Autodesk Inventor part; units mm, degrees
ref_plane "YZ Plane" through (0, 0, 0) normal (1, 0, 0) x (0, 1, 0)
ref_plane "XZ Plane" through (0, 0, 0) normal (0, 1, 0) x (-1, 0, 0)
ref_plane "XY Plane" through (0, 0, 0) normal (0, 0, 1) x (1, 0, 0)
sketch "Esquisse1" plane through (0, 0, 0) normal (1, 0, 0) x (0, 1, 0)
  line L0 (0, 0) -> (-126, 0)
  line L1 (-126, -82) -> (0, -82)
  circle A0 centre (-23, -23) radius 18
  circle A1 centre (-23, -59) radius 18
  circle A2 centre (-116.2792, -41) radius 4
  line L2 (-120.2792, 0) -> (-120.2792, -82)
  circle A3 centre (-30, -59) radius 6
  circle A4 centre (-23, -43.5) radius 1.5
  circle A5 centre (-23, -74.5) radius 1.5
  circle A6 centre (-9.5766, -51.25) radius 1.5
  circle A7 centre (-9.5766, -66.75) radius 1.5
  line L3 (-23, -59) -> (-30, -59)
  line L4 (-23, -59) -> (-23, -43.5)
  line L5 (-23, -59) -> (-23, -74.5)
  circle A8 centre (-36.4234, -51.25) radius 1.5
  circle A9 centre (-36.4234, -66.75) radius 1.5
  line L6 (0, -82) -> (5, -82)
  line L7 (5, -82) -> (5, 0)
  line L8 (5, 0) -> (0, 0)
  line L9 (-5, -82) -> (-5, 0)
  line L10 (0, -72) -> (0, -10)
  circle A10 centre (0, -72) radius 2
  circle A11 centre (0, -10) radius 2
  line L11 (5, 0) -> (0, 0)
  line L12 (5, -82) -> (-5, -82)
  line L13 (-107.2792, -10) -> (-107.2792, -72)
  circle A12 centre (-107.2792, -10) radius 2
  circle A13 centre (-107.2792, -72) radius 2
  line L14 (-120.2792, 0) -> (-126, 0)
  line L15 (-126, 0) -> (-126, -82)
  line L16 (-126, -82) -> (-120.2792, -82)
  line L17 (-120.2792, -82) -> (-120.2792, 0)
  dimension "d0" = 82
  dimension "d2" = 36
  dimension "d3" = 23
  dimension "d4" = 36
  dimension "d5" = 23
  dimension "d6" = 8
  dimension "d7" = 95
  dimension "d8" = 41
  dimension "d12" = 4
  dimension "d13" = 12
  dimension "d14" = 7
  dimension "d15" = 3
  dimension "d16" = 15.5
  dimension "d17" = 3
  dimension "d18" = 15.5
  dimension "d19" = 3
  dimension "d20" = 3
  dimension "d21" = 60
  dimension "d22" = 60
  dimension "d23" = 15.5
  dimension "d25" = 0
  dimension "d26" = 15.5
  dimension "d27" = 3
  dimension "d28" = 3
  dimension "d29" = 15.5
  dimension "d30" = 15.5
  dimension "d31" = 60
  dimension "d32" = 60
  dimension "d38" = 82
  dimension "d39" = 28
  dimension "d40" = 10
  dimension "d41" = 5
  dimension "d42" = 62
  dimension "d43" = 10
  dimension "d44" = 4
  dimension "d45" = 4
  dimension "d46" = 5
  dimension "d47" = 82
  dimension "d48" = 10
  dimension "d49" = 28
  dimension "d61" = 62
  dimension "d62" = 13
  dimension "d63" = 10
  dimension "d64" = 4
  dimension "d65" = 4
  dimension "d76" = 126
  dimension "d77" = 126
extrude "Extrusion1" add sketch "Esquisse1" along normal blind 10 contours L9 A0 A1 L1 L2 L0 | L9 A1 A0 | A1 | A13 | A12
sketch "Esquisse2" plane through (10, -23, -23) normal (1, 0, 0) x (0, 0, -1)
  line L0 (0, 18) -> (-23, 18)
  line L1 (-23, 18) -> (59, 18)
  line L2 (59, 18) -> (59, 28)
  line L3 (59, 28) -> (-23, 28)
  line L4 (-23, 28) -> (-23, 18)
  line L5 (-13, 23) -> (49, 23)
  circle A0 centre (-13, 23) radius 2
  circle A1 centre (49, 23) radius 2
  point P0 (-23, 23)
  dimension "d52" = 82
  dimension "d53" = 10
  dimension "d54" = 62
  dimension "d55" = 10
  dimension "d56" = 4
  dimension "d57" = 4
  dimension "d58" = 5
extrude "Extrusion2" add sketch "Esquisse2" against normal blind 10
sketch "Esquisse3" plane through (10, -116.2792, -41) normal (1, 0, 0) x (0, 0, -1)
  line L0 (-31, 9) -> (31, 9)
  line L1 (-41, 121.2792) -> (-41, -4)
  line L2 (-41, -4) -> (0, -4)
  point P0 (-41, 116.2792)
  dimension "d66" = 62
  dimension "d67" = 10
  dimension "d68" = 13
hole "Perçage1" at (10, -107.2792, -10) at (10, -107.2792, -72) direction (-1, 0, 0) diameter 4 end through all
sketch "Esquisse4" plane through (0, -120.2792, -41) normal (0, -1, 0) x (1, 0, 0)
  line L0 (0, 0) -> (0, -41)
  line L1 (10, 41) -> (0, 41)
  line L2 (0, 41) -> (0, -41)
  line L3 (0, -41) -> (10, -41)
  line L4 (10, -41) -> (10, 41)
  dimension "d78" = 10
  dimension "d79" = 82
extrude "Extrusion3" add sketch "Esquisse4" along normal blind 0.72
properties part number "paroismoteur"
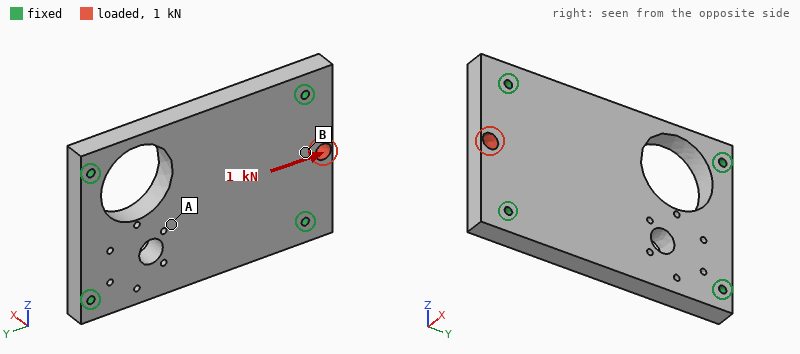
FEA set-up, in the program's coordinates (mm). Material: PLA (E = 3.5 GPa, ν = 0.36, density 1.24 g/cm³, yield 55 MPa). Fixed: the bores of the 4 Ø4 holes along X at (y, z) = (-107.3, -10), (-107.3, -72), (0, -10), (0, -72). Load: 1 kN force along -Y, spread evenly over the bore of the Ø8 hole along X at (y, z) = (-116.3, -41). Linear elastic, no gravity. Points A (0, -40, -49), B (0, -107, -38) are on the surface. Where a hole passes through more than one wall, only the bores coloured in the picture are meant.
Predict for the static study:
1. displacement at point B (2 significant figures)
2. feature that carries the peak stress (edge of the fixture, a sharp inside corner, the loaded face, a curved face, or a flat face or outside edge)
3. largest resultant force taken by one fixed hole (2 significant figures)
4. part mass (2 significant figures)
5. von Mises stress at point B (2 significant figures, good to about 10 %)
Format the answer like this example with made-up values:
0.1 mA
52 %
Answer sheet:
39 µm
a flat face or outside edge
410 N
110 g
4.2 MPa
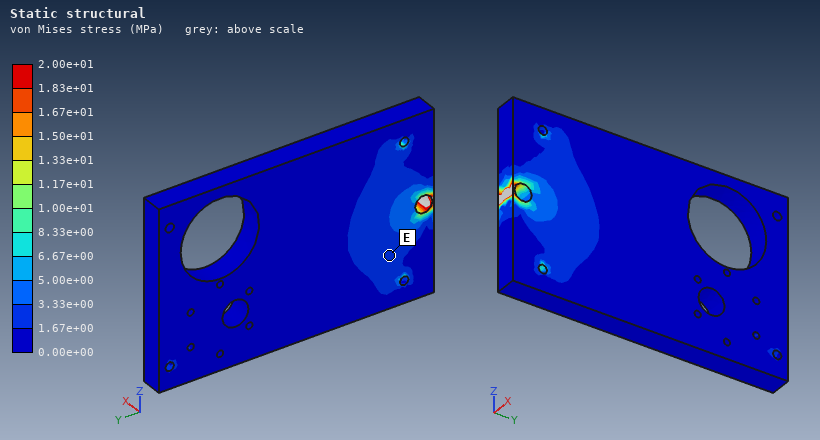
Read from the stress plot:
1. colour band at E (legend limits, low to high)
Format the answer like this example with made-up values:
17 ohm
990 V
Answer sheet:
1.67e+00 to 3.33e+00 MPa
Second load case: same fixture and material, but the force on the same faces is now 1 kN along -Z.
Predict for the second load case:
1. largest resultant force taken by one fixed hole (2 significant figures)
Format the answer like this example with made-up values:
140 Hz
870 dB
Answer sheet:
510 N
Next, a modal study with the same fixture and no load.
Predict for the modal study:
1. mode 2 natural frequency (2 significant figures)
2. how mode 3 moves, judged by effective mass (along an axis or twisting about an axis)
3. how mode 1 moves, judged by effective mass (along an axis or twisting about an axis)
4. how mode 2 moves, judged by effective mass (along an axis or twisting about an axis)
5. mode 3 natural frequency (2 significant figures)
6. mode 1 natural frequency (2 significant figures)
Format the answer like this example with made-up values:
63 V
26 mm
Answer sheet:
1600 Hz
twisting about Z
along X
twisting about Y
2800 Hz
1100 Hz
